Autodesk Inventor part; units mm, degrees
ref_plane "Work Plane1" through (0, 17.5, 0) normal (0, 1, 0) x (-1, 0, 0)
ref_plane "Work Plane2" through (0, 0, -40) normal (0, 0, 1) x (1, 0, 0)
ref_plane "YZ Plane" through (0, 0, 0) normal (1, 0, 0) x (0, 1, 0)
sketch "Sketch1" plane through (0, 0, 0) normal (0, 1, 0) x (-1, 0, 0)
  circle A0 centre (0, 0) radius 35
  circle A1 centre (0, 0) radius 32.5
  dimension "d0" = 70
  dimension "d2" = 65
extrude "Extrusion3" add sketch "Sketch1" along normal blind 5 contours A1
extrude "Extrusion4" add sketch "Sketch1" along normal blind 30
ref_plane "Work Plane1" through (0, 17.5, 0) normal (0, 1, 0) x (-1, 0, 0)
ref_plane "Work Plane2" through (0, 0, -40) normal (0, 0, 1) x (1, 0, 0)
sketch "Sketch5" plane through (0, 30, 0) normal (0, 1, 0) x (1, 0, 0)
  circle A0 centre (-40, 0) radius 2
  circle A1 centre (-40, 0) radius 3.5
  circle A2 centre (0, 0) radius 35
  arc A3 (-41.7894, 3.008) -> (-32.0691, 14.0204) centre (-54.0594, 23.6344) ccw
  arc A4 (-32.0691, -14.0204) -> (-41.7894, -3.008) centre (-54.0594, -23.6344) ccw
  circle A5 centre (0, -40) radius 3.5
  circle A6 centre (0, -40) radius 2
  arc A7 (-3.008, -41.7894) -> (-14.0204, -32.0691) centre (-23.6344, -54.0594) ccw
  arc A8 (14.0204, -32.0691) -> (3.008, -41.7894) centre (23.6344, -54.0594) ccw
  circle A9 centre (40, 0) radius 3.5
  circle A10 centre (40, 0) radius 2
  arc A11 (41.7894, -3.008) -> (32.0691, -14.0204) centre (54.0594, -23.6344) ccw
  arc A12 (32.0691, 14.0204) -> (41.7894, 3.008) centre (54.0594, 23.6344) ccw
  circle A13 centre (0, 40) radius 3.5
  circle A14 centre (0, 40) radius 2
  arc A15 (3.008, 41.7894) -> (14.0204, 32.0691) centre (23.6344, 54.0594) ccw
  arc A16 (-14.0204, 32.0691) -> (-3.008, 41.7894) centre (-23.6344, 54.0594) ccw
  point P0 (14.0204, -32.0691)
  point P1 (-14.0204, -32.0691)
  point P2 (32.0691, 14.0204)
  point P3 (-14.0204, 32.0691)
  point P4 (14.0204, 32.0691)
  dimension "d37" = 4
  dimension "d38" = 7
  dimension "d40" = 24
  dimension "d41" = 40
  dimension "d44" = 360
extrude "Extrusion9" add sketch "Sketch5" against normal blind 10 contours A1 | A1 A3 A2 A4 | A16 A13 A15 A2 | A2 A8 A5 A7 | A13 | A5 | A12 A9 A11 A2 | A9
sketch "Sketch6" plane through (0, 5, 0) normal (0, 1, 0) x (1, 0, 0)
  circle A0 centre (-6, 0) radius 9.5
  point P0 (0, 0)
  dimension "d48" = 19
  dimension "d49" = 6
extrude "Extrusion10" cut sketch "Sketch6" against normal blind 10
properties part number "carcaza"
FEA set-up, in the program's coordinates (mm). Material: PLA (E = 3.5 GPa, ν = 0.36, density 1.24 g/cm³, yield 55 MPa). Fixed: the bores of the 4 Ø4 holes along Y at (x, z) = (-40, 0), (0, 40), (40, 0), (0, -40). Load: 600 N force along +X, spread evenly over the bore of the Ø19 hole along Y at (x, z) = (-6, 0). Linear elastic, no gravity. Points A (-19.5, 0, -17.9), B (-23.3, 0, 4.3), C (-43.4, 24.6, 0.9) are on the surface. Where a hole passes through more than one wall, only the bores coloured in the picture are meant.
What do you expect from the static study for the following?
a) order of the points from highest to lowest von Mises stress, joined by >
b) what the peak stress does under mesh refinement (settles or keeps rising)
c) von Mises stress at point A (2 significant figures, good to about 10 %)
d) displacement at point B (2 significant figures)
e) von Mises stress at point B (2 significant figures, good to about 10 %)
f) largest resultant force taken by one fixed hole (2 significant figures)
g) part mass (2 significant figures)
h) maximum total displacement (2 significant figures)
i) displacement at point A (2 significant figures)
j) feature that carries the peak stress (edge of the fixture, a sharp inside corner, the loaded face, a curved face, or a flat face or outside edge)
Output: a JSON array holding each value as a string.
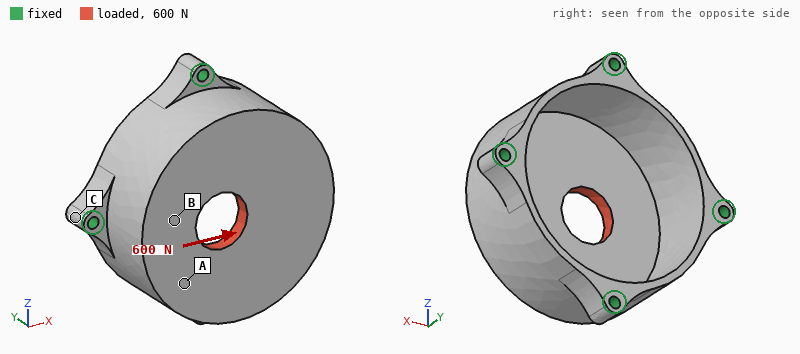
["B > A > C", "keeps rising", "1.6 MPa", "86 µm", "2.9 MPa", "210 N", "43 g", "91 µm", "76 µm", "edge of the fixture"]
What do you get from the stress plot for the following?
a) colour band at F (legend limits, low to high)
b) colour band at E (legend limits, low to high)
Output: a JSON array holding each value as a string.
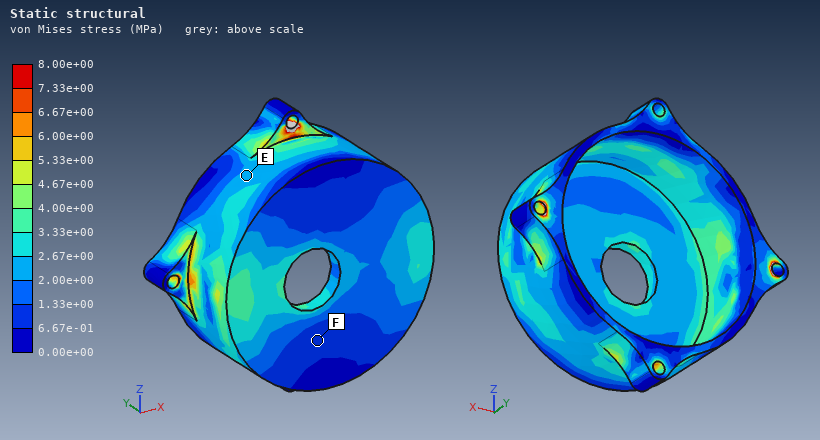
["6.67e-01 to 1.33e+00 MPa", "2.00e+00 to 2.67e+00 MPa"]
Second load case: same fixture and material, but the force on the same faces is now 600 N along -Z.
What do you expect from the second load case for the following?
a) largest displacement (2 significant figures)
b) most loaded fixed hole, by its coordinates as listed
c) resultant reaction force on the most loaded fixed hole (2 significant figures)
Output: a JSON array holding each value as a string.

["88 µm", "(-40, 0)", "240 N"]
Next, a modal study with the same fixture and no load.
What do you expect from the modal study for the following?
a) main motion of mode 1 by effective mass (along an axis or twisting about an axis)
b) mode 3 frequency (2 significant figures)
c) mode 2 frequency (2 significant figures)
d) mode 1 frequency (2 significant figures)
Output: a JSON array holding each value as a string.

["along Y", "2800 Hz", "2800 Hz", "2200 Hz"]
